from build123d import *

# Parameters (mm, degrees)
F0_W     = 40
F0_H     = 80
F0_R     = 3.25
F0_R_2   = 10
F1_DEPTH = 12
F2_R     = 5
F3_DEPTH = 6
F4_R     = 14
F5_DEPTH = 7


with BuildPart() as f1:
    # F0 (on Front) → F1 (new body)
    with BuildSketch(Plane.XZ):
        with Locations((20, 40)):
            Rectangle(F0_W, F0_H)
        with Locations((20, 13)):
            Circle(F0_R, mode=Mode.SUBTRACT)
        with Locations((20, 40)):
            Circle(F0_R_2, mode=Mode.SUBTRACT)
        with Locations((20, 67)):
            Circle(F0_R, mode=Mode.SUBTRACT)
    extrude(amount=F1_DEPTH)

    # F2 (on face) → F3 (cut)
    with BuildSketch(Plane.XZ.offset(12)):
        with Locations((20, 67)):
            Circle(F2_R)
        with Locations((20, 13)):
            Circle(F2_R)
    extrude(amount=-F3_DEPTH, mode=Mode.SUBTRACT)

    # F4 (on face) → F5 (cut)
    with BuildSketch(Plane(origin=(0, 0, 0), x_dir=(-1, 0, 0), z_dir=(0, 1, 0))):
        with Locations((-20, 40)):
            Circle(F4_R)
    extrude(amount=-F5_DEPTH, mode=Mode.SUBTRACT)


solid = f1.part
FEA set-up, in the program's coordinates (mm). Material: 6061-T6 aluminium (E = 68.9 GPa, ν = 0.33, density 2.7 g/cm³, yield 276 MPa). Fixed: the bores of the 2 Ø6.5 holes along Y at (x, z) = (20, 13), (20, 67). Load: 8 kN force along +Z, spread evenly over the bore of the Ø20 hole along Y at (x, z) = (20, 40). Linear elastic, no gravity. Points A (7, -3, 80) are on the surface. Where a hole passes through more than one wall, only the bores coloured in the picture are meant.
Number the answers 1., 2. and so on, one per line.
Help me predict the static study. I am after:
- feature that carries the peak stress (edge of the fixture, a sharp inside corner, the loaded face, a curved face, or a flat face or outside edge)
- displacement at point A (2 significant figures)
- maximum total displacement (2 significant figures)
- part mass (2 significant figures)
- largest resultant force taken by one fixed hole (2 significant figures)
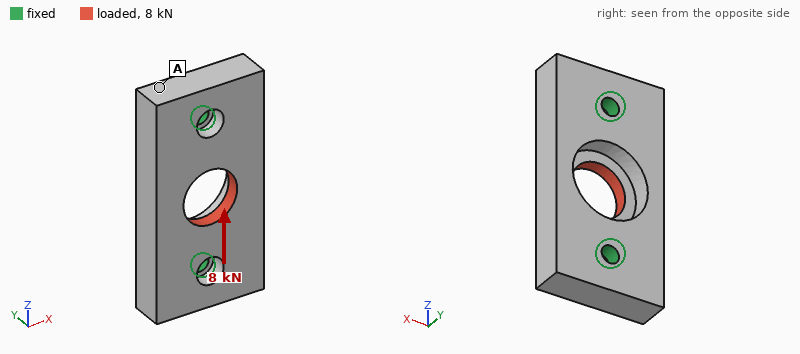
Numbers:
1. edge of the fixture
2. 7.5 µm
3. 14 µm
4. 84 g
5. 4.1 kN
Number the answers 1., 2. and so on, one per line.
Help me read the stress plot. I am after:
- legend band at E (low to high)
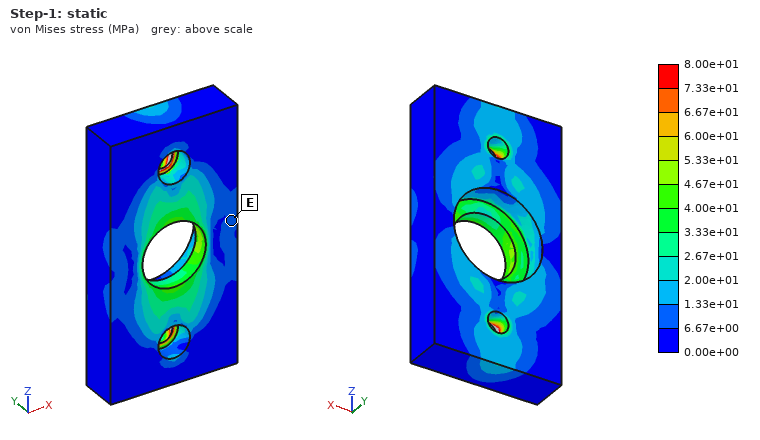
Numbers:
1. 6.67e+00 to 1.33e+01 MPa
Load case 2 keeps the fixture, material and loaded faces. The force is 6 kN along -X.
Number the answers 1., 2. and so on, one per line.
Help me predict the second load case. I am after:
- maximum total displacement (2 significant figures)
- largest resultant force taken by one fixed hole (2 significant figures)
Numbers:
1. 43 µm
2. 3.0 kN
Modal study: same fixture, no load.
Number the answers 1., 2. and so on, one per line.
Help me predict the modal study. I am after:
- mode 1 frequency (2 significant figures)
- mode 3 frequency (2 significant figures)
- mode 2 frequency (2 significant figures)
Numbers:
1. 7100 Hz
2. 11 kHz
3. 11 kHz
